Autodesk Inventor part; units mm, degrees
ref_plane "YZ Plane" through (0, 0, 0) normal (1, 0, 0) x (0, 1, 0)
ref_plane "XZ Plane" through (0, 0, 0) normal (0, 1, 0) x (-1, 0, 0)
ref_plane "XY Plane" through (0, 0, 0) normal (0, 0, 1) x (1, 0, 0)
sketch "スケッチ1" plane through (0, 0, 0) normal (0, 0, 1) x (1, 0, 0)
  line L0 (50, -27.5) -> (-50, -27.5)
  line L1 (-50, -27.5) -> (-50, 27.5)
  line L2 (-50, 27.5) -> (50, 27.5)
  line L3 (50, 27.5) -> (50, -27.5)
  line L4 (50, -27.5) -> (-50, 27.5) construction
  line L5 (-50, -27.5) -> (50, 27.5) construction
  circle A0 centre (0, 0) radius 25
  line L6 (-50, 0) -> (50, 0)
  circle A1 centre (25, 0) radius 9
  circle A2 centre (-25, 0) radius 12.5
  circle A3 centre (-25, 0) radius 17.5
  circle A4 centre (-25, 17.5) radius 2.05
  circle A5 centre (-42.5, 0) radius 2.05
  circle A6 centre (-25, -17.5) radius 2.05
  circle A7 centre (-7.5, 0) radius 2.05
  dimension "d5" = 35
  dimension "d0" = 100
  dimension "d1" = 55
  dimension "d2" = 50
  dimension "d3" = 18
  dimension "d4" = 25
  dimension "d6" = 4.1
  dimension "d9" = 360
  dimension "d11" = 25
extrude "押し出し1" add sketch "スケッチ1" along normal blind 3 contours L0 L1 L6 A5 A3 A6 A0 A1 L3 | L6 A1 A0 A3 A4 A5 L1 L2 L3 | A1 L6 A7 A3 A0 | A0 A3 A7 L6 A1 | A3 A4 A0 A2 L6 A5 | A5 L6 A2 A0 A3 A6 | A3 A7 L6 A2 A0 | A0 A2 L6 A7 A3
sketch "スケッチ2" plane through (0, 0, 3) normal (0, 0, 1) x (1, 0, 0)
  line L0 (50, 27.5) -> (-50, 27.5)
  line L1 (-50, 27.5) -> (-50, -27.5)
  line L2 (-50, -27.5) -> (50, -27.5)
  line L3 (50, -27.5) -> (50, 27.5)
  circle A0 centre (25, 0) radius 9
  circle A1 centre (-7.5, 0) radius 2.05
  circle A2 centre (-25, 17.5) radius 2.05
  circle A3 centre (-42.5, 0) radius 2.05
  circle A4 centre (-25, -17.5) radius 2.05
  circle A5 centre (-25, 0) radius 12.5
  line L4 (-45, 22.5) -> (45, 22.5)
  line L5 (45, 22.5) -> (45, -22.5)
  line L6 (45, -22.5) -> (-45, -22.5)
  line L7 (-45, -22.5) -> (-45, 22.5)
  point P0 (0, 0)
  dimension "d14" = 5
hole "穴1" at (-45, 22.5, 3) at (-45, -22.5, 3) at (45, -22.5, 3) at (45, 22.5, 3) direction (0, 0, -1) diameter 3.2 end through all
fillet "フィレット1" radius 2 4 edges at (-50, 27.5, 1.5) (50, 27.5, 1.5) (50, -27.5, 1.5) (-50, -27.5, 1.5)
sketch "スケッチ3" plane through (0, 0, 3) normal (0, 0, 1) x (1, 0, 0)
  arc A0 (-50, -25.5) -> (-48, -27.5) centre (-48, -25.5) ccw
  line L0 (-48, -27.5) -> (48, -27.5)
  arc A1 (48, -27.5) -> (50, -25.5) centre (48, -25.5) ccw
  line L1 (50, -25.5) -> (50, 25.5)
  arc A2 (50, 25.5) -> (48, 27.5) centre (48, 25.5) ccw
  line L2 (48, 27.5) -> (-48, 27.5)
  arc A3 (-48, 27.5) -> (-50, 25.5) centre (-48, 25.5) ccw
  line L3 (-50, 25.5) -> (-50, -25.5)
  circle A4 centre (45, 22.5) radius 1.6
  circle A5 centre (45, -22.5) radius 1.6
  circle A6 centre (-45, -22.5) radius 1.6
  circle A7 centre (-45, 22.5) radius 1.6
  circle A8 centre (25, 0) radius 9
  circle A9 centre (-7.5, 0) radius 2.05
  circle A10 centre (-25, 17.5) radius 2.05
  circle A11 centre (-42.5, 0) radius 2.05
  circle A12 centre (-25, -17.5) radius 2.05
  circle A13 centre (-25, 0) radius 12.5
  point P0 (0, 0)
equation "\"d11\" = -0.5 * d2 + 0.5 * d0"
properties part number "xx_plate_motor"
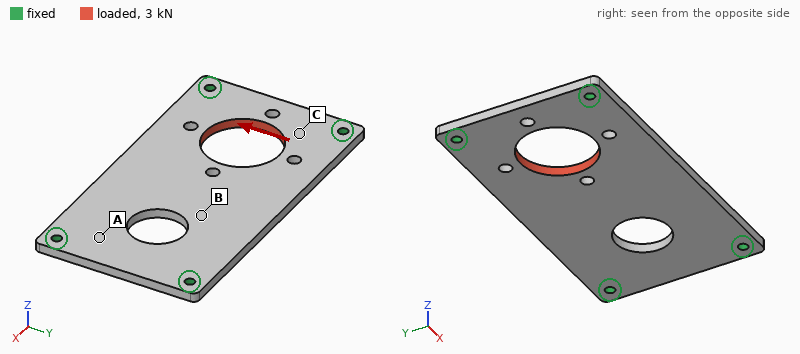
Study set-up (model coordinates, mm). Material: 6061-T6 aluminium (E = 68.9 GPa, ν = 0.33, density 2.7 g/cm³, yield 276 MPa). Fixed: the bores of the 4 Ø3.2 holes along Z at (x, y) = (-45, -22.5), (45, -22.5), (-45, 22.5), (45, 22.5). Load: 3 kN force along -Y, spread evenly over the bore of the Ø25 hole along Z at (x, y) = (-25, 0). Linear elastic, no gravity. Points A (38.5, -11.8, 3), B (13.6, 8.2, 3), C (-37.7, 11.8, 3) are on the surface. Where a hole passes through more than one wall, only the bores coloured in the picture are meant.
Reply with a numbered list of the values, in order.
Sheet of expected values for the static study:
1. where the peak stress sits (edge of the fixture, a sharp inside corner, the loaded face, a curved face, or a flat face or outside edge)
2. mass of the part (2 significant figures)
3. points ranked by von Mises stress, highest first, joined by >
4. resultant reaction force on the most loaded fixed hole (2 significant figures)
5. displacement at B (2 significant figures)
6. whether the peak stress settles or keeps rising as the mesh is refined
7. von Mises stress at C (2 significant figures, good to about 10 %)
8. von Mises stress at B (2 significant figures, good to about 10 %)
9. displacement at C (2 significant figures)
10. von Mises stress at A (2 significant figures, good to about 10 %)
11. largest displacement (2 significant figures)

1. edge of the fixture
2. 38 g
3. C > B > A
4. 1.1 kN
5. 19 µm
6. keeps rising
7. 23 MPa
8. 14 MPa
9. 10 µm
10. 6.8 MPa
11. 31 µm
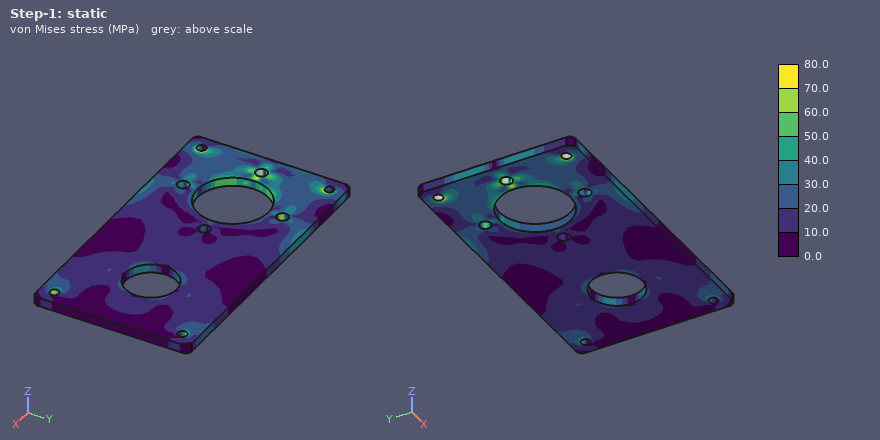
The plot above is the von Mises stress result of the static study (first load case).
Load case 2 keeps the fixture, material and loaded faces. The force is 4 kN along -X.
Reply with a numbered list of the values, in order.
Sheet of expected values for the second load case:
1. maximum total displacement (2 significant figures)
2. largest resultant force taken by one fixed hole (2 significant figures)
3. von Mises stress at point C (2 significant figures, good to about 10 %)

1. 24 µm
2. 1.4 kN
3. 22 MPa
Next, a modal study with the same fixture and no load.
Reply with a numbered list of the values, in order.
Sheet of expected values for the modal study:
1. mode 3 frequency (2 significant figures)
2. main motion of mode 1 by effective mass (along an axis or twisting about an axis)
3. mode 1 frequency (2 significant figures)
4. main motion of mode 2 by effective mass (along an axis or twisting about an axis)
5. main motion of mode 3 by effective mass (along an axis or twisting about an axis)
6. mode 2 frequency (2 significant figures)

1. 4700 Hz
2. along Z
3. 1700 Hz
4. twisting about X
5. twisting about Y
6. 2600 Hz
